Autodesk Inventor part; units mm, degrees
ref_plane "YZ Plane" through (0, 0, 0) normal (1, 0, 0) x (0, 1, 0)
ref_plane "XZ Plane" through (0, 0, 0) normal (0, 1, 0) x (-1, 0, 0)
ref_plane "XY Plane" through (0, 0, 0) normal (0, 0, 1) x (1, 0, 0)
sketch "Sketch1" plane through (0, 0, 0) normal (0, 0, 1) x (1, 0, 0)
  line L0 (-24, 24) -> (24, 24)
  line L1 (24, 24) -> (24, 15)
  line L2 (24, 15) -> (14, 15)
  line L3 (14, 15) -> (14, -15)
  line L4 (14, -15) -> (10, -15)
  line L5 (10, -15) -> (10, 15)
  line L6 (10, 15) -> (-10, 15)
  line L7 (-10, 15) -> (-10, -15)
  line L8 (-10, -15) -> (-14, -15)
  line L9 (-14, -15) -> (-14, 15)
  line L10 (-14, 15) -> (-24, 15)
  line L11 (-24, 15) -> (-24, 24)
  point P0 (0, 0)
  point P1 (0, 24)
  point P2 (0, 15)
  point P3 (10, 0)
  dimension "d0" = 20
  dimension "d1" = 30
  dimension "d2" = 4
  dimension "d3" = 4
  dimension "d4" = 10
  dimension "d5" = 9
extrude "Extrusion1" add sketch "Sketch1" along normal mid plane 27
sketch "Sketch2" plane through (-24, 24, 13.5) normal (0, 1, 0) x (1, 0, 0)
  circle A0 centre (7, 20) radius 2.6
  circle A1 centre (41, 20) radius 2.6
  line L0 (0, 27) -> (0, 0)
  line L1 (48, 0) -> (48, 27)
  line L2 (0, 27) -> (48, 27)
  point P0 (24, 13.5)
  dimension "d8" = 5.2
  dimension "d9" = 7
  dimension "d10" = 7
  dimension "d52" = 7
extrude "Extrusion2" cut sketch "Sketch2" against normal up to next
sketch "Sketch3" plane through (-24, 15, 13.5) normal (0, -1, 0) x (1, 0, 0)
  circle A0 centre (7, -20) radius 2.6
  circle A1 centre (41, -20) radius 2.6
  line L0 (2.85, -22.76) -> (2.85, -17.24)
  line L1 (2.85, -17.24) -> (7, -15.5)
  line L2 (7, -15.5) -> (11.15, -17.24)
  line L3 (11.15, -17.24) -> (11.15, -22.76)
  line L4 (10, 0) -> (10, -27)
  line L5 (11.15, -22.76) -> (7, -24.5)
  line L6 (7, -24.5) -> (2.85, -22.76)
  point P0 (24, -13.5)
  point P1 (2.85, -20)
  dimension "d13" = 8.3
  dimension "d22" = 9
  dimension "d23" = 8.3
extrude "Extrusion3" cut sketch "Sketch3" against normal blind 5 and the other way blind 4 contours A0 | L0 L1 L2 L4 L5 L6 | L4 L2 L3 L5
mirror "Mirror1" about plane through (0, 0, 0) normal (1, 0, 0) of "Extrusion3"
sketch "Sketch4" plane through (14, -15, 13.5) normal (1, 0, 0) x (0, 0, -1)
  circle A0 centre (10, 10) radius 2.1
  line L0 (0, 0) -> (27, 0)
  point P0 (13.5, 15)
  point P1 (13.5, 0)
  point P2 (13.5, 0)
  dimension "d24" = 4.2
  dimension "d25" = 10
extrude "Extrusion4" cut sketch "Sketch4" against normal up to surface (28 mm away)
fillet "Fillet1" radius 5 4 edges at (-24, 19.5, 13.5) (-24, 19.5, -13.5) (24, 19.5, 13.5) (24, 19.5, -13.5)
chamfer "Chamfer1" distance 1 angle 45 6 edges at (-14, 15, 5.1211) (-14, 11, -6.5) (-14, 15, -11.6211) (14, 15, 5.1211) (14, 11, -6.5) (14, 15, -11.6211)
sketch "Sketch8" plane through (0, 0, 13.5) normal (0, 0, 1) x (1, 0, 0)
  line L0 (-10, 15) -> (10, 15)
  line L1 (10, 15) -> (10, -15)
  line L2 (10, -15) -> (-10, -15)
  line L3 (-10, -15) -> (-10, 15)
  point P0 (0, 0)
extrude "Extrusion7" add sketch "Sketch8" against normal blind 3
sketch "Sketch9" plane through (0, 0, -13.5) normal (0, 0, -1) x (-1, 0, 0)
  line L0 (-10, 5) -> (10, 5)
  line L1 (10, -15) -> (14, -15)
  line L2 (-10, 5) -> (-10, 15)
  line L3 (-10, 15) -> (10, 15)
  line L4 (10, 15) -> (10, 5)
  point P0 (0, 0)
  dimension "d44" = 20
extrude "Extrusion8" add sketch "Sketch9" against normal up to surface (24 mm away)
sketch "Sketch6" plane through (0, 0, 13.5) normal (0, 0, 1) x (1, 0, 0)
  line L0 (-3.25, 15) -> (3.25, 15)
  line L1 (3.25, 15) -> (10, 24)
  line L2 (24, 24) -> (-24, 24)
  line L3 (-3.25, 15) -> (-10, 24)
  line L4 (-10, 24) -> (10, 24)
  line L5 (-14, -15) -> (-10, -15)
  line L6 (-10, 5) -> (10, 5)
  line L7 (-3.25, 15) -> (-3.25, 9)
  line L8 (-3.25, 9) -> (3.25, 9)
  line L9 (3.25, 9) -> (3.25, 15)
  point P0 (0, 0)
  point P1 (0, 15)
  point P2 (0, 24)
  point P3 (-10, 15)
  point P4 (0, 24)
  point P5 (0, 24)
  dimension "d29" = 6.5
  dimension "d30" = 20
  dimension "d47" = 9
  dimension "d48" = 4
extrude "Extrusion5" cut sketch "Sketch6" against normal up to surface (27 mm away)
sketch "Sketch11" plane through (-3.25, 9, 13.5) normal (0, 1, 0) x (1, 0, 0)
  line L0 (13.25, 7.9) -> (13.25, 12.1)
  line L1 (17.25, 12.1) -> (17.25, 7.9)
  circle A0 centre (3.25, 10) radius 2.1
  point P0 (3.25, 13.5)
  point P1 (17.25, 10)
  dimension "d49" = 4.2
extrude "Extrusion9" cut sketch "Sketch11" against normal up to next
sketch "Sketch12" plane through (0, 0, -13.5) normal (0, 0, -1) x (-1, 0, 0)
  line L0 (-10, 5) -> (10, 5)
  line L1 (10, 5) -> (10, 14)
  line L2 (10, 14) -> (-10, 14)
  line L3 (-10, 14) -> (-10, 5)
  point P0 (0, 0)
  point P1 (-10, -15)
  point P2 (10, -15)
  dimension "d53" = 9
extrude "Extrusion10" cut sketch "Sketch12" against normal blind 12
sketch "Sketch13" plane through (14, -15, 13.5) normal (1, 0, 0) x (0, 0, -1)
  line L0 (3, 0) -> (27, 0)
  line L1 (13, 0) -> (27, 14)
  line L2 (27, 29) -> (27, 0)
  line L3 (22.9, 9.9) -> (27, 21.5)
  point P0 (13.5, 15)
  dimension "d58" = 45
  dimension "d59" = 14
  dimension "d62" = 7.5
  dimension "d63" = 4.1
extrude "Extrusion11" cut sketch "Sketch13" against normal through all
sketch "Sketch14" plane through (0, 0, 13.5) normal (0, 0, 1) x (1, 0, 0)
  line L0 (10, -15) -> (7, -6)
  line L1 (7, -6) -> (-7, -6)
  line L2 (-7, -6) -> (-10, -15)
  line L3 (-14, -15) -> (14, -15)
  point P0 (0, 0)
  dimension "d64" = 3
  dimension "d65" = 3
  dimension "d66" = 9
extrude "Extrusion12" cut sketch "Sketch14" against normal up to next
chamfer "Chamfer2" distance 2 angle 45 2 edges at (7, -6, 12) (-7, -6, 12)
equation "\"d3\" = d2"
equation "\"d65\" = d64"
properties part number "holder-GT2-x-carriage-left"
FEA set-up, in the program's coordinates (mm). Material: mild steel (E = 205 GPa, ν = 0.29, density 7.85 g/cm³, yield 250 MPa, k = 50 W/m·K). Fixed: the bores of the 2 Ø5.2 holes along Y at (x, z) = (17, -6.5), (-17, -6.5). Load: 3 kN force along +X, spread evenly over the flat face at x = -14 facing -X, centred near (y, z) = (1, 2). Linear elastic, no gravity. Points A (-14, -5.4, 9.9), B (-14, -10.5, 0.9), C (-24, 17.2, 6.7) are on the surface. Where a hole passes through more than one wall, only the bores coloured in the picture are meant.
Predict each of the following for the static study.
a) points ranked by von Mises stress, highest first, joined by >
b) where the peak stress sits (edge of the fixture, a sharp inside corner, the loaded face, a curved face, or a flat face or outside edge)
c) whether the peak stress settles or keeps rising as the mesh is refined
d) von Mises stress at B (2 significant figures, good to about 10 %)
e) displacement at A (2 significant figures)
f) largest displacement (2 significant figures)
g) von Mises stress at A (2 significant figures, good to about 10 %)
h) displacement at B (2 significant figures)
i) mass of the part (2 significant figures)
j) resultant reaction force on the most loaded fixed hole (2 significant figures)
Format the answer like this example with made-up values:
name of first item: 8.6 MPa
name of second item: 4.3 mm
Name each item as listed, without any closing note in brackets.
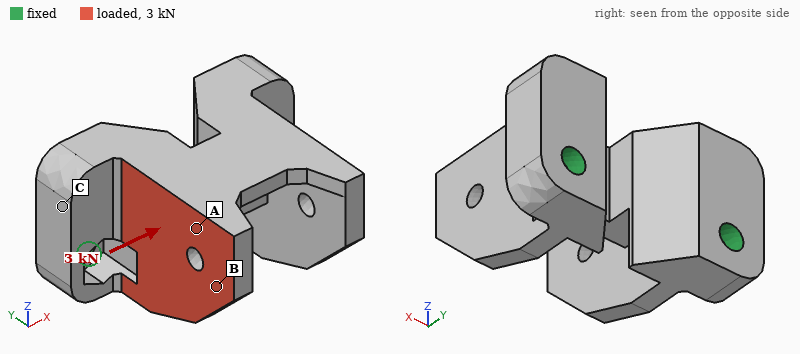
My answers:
points ranked by von Mises stress, highest first, joined by >: A > B > C
where the peak stress sits: edge of the fixture
whether the peak stress settles or keeps rising as the mesh is refined: keeps rising
von Mises stress at B: 56 MPa
displacement at A: 34 µm
largest displacement: 85 µm
von Mises stress at A: 100 MPa
displacement at B: 70 µm
mass of the part: 130 g
resultant reaction force on the most loaded fixed hole: 2.3 kN
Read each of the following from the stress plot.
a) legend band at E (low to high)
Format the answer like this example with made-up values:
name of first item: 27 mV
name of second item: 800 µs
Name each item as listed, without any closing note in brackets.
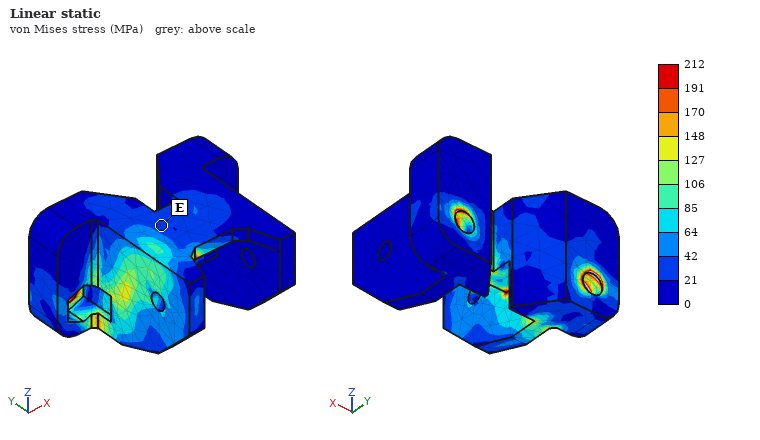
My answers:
legend band at E: 21 to 42 MPa
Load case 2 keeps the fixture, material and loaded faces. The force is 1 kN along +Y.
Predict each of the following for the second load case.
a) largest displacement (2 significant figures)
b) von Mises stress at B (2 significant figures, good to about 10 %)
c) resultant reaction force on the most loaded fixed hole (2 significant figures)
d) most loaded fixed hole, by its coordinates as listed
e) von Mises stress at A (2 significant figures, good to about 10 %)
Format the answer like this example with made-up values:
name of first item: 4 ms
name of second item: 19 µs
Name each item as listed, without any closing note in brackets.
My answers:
largest displacement: 19 µm
von Mises stress at B: 6.2 MPa
resultant reaction force on the most loaded fixed hole: 930 N
most loaded fixed hole, by its coordinates as listed: (-17, -6.5)
von Mises stress at A: 14 MPa
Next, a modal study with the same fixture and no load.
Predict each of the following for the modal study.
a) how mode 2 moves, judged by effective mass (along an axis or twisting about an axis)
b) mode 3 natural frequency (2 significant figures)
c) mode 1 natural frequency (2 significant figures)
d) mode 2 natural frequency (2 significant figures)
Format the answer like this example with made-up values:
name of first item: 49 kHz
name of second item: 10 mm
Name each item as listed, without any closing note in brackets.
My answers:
how mode 2 moves, judged by effective mass: along X
mode 3 natural frequency: 10 kHz
mode 1 natural frequency: 3900 Hz
mode 2 natural frequency: 6300 Hz
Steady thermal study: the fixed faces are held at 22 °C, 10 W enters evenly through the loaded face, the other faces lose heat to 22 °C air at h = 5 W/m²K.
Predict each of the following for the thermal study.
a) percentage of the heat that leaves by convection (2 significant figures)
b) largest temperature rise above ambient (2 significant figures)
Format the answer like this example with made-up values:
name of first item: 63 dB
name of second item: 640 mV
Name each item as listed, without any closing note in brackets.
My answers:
percentage of the heat that leaves by convection: 3.3 %
largest temperature rise above ambient: 31 K
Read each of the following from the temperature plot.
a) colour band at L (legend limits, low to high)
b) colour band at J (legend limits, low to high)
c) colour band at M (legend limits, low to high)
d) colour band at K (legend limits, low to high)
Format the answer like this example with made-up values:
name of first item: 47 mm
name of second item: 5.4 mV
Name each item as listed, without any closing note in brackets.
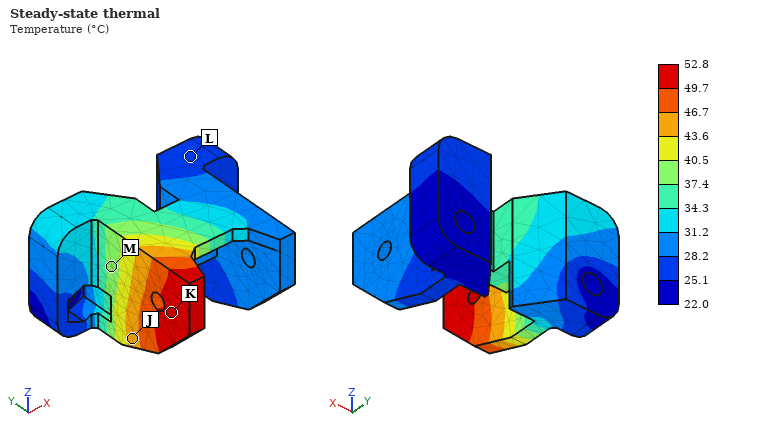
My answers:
colour band at L: 25.1 to 28.2 °C
colour band at J: 43.6 to 46.7 °C
colour band at M: 37.4 to 40.5 °C
colour band at K: 49.7 to 52.8 °C
